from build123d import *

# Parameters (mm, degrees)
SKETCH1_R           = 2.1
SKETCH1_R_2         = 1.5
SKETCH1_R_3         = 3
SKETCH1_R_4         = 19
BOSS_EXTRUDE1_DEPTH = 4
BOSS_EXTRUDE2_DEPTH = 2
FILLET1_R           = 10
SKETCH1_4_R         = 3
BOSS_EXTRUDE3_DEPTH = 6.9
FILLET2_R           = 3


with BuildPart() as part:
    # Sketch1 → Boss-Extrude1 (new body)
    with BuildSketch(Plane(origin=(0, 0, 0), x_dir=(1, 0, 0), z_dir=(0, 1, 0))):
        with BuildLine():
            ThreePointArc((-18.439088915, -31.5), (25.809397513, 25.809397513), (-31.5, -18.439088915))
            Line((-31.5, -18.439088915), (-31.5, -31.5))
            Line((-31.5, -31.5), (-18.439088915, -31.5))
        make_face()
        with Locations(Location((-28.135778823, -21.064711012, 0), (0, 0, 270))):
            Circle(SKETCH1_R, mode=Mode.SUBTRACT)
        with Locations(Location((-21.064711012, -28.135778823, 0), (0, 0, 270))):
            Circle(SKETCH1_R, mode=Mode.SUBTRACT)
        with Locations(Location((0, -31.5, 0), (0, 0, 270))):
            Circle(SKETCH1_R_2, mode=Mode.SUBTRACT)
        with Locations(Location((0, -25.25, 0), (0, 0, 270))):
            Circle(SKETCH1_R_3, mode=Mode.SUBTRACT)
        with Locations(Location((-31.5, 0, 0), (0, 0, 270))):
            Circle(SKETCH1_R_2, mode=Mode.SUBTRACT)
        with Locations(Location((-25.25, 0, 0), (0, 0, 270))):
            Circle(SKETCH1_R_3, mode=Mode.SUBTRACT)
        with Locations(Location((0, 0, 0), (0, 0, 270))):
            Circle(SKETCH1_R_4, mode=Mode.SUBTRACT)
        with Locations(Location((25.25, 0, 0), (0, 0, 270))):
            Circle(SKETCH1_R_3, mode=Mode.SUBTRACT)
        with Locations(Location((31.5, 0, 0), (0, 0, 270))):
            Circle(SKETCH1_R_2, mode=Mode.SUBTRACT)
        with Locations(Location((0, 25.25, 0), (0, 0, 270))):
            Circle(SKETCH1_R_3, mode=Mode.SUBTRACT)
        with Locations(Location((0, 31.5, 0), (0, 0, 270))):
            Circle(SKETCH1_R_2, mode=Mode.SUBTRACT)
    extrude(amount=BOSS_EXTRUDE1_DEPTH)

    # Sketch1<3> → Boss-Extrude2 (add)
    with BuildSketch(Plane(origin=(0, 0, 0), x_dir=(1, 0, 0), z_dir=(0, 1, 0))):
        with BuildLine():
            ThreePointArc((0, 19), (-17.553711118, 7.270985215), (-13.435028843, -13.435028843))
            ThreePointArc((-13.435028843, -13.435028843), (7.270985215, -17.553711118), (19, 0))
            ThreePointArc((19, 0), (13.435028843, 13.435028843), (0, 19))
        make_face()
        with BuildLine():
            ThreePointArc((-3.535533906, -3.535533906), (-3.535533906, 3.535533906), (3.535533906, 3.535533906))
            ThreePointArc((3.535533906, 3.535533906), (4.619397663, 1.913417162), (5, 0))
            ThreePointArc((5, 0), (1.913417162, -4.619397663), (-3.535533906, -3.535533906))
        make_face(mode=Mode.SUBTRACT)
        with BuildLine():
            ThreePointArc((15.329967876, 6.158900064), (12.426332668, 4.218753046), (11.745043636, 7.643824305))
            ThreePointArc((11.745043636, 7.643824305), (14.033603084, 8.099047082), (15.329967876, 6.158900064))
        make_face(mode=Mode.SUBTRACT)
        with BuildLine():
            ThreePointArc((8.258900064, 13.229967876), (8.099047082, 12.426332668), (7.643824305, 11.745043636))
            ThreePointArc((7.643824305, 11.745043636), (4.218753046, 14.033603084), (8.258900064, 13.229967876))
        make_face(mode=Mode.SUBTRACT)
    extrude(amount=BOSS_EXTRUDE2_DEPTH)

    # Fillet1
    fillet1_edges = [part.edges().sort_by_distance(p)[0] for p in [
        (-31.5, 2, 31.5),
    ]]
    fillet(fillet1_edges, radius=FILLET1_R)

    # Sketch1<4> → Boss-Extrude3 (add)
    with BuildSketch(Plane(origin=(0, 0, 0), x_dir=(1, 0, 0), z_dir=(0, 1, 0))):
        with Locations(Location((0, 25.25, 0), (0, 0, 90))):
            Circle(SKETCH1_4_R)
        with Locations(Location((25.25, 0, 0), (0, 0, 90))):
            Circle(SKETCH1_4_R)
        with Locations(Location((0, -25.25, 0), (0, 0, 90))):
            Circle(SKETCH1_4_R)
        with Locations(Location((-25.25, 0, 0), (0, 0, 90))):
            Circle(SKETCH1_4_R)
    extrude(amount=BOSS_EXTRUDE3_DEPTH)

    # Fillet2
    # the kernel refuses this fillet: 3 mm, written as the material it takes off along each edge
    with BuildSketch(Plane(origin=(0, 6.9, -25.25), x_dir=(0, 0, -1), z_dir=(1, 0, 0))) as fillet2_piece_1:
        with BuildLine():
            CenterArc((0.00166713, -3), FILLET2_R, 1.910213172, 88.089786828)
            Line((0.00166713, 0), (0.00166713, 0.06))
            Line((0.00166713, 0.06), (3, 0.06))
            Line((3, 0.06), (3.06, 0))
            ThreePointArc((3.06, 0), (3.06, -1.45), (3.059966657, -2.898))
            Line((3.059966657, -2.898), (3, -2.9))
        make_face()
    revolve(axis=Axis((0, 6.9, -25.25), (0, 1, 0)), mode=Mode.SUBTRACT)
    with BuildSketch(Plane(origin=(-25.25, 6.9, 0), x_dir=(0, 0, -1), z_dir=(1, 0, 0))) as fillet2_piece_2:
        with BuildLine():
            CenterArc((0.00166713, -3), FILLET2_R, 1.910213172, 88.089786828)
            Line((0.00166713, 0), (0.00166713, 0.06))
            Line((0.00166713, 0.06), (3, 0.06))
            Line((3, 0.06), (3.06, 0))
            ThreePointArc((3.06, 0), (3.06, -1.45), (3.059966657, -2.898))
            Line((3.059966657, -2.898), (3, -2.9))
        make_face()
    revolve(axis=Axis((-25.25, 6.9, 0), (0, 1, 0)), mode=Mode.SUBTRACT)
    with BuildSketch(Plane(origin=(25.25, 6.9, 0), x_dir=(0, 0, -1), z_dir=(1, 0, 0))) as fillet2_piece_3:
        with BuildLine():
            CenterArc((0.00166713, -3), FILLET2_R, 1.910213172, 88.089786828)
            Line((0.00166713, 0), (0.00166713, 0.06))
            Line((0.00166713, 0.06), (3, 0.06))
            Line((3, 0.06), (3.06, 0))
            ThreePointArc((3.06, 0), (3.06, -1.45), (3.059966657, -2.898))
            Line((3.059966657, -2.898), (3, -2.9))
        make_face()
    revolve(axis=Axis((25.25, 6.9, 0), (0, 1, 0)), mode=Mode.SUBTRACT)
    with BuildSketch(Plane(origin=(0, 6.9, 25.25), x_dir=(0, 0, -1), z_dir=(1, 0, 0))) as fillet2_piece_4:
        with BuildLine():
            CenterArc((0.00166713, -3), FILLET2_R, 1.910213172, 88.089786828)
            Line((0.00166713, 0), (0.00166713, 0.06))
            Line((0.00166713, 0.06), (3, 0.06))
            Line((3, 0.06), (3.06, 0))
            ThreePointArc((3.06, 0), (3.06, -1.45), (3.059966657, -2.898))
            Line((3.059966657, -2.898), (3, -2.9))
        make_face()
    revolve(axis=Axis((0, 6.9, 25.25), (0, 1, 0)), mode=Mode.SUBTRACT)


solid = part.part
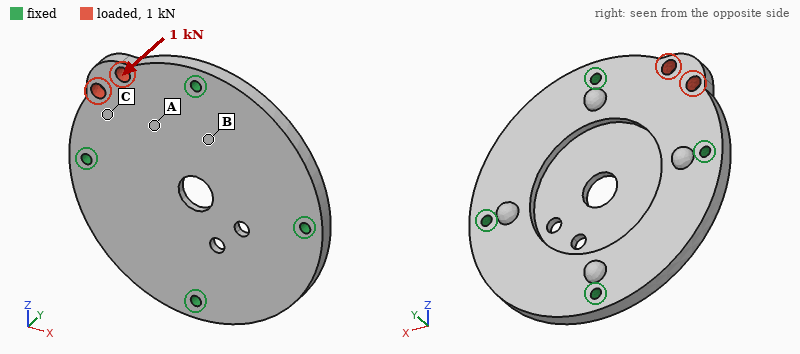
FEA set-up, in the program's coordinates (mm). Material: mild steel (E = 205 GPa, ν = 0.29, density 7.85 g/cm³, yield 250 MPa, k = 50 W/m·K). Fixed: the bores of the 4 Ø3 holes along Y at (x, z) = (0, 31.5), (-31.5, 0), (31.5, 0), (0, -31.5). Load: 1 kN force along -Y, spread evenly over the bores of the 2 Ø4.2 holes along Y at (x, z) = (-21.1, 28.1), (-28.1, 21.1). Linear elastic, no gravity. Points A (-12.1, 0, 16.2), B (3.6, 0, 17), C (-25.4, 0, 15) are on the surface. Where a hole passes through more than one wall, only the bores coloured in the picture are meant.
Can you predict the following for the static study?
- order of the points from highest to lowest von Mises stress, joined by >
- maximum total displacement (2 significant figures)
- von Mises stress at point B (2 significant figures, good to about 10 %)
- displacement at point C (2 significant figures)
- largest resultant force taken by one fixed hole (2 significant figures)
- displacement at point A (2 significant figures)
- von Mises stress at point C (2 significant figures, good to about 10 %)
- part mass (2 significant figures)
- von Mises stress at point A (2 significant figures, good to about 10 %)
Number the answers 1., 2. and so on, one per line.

1. C > A > B
2. 93 µm
3. 26 MPa
4. 36 µm
5. 580 N
6. 15 µm
7. 100 MPa
8. 110 g
9. 67 MPa
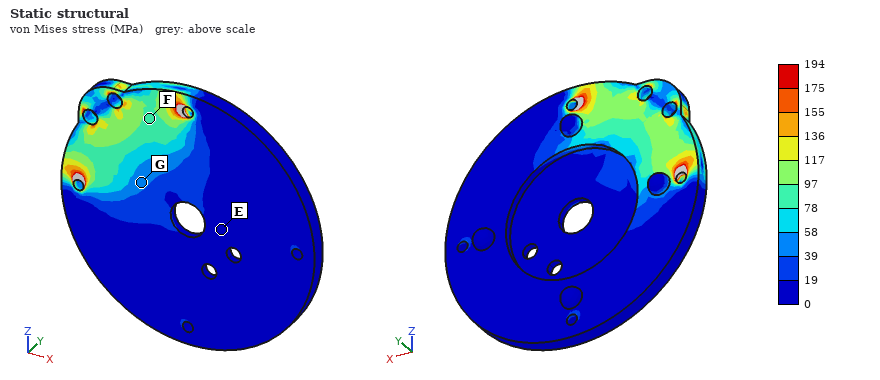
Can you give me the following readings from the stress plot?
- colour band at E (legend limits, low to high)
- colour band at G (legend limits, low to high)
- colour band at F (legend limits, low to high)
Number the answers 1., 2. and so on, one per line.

1. 0 to 19 MPa
2. 39 to 58 MPa
3. 78 to 97 MPa
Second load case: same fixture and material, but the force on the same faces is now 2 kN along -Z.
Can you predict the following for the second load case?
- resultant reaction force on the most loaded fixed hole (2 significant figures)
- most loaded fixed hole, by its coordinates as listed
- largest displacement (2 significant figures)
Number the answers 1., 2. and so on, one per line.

1. 1.3 kN
2. (-31.5, 0)
3. 5.3 µm
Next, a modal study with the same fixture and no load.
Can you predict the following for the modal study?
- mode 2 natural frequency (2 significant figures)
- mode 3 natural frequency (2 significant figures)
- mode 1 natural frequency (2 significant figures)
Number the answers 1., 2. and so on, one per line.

1. 7400 Hz
2. 8000 Hz
3. 7200 Hz
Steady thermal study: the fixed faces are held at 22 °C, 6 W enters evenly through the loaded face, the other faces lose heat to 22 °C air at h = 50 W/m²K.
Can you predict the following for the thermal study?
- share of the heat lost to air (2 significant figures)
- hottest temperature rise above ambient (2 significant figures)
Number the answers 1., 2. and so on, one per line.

1. 23 %
2. 24 K
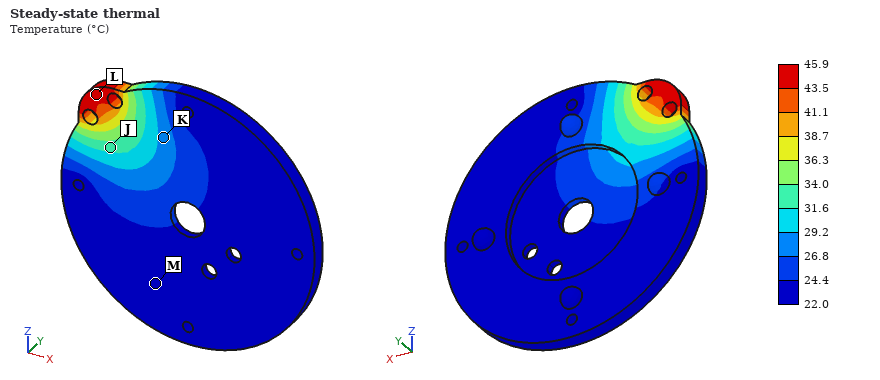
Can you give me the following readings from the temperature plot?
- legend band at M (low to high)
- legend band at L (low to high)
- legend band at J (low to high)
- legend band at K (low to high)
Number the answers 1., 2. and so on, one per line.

1. 22.0 to 24.4 °C
2. 43.5 to 45.9 °C
3. 31.6 to 34.0 °C
4. 26.8 to 29.2 °C
